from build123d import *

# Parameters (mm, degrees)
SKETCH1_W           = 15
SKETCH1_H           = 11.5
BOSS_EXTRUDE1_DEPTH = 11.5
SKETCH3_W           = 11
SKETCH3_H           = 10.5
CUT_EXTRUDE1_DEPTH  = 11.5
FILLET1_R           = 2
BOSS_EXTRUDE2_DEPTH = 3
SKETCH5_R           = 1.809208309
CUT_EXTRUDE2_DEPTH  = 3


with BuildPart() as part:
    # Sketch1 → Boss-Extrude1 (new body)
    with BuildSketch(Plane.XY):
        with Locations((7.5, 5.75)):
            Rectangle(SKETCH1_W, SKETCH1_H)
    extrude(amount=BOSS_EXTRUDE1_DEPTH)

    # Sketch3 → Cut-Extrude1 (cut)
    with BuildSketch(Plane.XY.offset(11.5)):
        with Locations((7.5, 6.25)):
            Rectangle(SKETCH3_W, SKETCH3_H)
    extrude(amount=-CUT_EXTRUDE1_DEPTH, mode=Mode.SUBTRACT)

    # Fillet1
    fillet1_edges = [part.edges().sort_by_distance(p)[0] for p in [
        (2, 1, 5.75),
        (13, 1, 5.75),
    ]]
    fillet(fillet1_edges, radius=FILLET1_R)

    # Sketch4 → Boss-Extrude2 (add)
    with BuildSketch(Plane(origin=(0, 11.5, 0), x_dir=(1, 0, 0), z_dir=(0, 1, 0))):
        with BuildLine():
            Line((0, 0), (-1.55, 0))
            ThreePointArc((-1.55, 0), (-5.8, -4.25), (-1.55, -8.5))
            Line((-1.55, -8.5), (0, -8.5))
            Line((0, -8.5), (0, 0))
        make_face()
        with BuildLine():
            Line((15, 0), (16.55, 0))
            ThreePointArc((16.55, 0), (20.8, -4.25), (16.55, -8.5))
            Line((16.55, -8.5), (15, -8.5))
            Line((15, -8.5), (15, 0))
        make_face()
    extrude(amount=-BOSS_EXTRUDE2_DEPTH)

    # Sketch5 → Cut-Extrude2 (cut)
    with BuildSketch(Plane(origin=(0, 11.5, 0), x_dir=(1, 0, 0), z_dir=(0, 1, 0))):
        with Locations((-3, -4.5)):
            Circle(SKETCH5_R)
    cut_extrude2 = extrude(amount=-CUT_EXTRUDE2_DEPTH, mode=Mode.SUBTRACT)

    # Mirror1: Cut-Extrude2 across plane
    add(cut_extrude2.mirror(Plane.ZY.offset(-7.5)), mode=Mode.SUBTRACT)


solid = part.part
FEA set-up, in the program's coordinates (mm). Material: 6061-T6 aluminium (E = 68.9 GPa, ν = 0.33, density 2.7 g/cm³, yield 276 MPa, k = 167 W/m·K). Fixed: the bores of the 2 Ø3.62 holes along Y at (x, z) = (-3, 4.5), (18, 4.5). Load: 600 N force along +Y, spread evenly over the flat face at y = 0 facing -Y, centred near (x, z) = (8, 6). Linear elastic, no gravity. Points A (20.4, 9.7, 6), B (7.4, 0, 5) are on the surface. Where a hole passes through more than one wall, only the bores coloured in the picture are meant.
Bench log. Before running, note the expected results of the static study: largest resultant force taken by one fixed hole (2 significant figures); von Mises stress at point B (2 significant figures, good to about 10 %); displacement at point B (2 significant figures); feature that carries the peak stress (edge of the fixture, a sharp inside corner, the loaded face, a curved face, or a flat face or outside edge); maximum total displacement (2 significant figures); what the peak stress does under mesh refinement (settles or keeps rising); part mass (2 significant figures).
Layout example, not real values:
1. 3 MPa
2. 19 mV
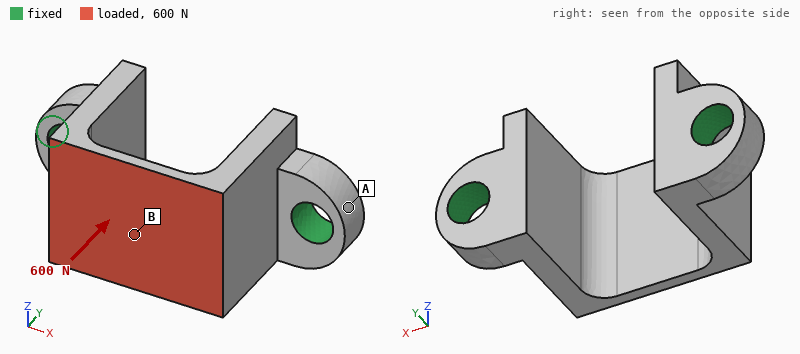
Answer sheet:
1. 320 N
2. 88 MPa
3. 25 µm
4. edge of the fixture
5. 32 µm
6. keeps rising
7. 2.3 g
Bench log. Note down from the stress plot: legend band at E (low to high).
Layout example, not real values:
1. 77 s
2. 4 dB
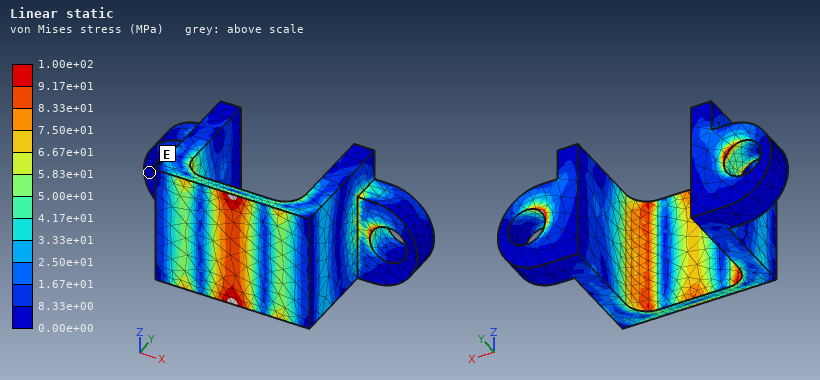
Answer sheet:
1. 0.00e+00 to 8.33e+00 MPa
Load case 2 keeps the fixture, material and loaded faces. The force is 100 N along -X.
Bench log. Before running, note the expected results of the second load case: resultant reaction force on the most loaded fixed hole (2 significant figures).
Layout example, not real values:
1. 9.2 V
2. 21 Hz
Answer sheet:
1. 58 N
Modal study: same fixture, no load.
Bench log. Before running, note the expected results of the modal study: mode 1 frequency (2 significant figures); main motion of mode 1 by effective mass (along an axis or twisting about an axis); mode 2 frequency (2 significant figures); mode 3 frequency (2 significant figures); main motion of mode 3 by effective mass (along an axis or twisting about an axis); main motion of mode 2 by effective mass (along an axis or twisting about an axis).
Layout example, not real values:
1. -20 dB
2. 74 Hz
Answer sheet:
1. 14 kHz
2. along X
3. 17 kHz
4. 21 kHz
5. twisting about Y
6. along Z
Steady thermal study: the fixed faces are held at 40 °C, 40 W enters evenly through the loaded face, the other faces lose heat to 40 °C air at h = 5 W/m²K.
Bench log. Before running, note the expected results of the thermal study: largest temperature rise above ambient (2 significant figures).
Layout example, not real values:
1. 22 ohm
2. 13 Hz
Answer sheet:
1. 78 K
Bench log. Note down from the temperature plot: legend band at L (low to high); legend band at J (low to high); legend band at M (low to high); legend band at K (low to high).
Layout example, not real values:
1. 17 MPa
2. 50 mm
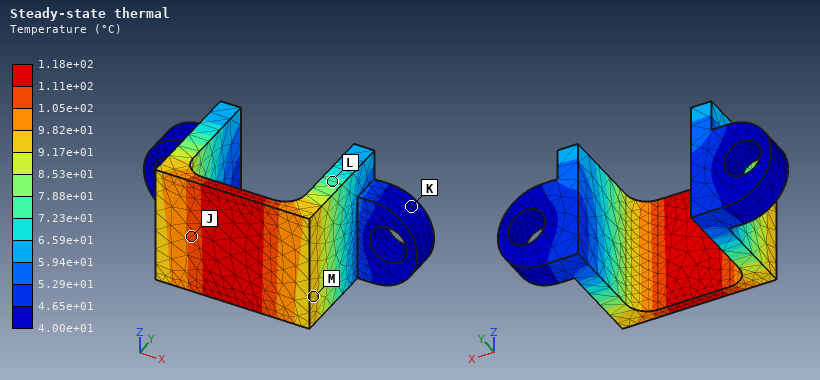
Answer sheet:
1. 7.23e+01 to 7.88e+01 °C
2. 1.05e+02 to 1.11e+02 °C
3. 9.17e+01 to 9.82e+01 °C
4. 4.00e+01 to 4.65e+01 °C
